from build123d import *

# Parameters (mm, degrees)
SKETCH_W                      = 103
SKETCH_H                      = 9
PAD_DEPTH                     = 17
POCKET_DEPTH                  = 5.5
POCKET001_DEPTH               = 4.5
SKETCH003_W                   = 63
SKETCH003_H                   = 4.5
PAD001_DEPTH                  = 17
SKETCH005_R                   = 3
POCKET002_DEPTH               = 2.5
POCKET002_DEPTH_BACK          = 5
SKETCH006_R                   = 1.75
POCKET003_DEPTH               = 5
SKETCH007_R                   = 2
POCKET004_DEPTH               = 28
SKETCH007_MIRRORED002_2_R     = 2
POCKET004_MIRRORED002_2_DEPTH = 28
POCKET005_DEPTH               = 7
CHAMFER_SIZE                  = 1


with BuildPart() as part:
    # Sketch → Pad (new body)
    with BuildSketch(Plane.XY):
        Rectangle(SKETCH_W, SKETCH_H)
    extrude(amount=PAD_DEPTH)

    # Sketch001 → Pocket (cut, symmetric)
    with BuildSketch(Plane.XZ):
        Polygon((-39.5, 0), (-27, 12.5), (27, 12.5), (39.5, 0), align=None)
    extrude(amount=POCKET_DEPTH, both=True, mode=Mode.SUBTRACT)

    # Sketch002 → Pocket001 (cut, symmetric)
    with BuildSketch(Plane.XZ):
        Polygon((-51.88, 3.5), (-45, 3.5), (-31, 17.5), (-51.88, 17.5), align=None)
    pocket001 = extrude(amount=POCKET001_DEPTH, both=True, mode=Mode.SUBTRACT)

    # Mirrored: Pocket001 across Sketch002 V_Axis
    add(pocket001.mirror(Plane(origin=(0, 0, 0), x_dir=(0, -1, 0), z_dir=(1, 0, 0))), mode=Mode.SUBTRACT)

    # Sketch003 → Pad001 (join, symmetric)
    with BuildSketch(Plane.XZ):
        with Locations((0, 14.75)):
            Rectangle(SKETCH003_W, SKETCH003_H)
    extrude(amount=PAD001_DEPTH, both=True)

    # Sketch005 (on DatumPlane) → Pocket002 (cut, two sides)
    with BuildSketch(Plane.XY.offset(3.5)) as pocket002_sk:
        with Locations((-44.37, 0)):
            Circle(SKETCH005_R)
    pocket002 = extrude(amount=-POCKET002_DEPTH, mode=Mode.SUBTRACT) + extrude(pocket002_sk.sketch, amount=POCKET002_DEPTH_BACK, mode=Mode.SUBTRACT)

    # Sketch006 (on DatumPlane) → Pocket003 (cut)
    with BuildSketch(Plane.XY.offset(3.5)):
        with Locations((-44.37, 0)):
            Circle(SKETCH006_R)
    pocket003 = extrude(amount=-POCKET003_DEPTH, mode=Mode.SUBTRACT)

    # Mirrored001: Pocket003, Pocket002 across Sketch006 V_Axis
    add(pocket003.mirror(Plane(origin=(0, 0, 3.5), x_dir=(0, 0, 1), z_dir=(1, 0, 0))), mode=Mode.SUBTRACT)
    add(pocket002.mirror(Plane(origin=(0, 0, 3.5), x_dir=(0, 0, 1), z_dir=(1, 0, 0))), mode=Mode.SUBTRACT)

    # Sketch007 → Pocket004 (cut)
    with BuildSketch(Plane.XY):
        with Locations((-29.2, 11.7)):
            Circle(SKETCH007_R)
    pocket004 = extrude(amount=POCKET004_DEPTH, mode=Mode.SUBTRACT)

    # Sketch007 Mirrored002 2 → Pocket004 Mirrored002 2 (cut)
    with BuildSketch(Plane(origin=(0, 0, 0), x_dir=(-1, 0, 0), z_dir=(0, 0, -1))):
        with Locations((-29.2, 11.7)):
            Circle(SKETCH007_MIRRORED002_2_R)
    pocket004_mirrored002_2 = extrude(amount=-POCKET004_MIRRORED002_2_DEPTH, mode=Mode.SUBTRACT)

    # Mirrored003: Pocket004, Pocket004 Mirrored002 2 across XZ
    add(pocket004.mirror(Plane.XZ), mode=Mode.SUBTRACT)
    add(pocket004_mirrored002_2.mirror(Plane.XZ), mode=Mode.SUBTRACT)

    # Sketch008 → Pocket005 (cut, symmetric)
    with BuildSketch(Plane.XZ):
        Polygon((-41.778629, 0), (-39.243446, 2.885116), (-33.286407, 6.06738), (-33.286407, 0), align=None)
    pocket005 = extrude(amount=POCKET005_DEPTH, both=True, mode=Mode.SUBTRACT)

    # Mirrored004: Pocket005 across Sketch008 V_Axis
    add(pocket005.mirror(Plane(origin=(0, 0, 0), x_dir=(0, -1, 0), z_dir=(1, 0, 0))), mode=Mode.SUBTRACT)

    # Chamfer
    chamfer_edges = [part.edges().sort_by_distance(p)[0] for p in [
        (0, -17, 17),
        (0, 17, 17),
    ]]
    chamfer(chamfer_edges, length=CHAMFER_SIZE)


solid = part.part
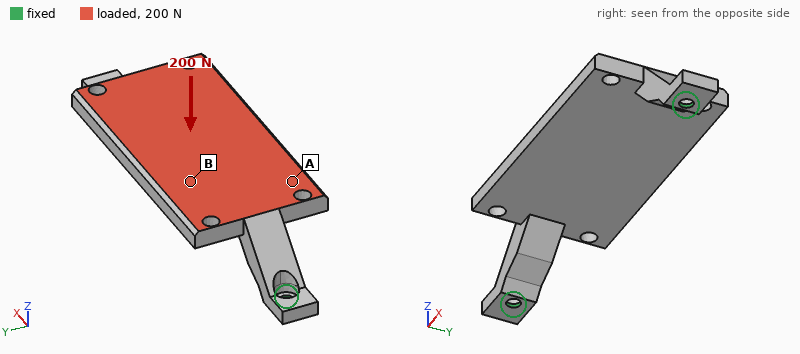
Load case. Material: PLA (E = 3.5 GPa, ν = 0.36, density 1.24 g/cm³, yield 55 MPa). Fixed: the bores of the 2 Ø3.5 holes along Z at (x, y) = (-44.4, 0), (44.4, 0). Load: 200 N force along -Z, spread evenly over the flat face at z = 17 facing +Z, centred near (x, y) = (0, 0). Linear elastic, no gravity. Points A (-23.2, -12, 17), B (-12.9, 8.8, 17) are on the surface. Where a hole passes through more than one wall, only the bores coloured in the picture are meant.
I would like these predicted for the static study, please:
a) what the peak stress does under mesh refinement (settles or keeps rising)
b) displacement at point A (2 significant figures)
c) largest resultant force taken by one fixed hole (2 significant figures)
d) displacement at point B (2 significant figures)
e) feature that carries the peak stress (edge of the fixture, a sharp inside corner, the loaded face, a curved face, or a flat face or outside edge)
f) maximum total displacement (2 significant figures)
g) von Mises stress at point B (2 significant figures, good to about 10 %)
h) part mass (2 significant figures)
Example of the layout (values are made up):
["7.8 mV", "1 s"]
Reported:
["keeps rising", "0.18 mm", "180 N", "0.30 mm", "edge of the fixture", "0.39 mm", "5.7 MPa", "14 g"]
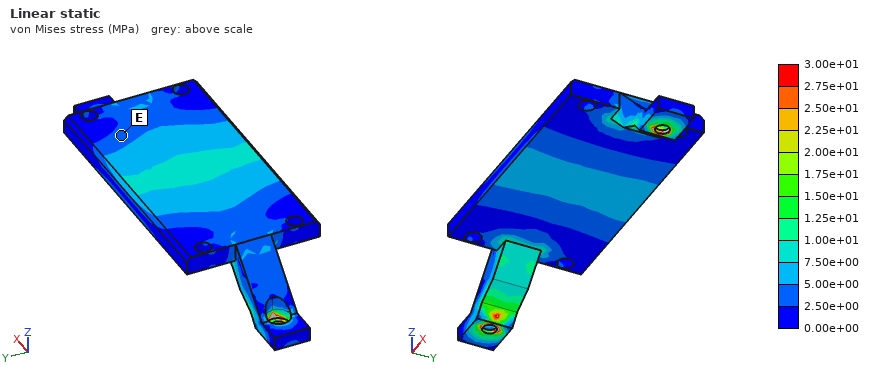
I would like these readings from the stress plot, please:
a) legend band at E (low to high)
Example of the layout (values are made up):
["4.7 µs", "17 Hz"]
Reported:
["2.50e+00 to 5.00e+00 MPa"]
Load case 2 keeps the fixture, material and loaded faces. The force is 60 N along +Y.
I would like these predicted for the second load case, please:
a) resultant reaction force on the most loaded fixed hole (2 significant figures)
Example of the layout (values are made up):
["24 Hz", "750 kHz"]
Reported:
["30 N"]
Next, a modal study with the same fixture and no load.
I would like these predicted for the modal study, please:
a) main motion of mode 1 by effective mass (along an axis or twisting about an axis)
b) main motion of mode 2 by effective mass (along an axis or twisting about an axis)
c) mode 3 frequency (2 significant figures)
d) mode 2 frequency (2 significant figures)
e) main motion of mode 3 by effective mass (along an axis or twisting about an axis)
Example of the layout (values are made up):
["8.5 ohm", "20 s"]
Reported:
["along Y", "along X", "1200 Hz", "1100 Hz", "along Z"]
